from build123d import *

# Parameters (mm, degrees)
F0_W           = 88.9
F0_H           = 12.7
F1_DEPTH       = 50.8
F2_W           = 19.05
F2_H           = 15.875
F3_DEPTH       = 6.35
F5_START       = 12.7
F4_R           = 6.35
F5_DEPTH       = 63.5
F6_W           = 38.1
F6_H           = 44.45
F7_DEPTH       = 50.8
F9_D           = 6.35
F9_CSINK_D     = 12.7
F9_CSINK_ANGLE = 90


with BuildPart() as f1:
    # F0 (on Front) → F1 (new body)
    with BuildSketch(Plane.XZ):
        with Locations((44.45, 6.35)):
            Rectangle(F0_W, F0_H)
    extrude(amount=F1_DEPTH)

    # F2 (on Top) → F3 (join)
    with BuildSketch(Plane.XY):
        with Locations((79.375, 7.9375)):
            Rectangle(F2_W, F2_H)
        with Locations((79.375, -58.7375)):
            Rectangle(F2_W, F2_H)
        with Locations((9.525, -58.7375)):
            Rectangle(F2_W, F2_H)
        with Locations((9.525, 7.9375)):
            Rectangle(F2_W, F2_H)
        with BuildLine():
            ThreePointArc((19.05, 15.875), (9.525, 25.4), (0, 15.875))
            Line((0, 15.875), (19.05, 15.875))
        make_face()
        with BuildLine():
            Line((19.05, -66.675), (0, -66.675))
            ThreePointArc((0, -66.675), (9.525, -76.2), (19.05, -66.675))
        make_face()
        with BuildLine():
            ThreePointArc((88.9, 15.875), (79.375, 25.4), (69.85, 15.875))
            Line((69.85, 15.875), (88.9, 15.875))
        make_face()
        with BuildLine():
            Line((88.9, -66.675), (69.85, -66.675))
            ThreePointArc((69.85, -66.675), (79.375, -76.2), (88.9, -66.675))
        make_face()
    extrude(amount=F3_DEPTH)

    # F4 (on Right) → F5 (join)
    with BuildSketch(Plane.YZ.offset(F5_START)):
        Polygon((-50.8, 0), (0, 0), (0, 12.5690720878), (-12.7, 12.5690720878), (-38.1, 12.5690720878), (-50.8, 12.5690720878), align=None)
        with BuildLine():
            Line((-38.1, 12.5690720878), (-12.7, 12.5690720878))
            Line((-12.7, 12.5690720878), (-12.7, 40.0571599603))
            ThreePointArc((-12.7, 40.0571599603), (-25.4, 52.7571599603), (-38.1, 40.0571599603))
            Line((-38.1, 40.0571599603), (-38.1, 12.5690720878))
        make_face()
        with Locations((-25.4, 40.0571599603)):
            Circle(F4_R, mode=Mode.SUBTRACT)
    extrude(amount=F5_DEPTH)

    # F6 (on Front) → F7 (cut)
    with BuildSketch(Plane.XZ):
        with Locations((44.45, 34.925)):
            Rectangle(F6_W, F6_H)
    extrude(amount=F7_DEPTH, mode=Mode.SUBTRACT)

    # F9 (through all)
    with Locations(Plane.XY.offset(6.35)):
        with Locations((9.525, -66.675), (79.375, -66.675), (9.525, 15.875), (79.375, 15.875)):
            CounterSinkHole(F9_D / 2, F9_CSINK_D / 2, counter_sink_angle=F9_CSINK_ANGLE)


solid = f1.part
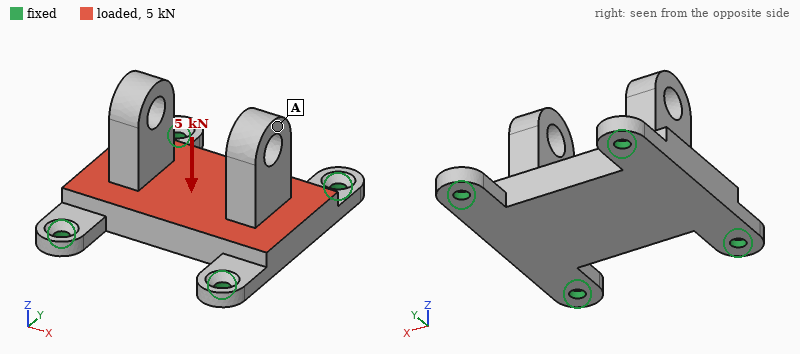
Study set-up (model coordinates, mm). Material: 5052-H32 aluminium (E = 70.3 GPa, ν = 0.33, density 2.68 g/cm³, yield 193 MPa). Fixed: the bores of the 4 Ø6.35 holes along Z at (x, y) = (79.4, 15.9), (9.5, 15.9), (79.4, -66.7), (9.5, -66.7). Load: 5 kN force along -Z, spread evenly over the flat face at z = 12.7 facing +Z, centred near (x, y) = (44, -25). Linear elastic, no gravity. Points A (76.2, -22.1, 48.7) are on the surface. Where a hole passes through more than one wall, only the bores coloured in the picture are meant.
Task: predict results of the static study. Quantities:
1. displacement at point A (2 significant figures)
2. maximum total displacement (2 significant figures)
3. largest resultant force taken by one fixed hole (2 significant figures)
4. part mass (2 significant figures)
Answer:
57 µm
66 µm
2.0 kN
240 g
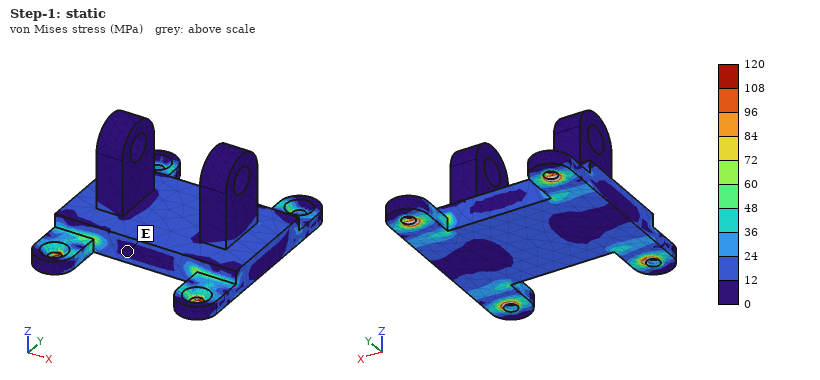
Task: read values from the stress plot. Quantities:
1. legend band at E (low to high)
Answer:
0 to 12 MPa
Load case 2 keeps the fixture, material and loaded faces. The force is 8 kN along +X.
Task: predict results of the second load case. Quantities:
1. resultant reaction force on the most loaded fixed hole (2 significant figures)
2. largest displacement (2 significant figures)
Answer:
2.4 kN
67 µm
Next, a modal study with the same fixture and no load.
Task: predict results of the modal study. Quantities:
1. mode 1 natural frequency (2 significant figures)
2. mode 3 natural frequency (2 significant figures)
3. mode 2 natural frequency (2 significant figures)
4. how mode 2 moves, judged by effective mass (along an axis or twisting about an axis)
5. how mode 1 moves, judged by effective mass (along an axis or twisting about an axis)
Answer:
3200 Hz
4600 Hz
3600 Hz
along X
along Z
